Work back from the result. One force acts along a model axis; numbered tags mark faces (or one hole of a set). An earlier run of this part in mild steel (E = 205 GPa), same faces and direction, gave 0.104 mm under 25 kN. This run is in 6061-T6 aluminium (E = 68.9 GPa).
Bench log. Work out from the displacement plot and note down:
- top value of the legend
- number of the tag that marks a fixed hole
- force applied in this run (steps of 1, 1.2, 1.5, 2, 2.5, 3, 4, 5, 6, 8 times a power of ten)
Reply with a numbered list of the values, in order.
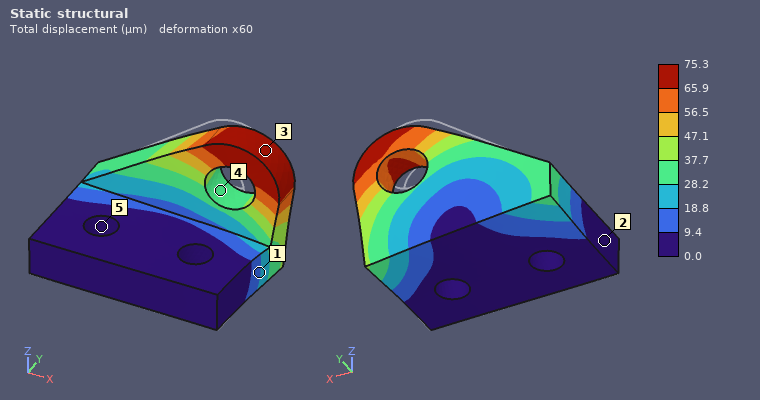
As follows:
1. 75.3 µm
2. 5
3. 6 kN
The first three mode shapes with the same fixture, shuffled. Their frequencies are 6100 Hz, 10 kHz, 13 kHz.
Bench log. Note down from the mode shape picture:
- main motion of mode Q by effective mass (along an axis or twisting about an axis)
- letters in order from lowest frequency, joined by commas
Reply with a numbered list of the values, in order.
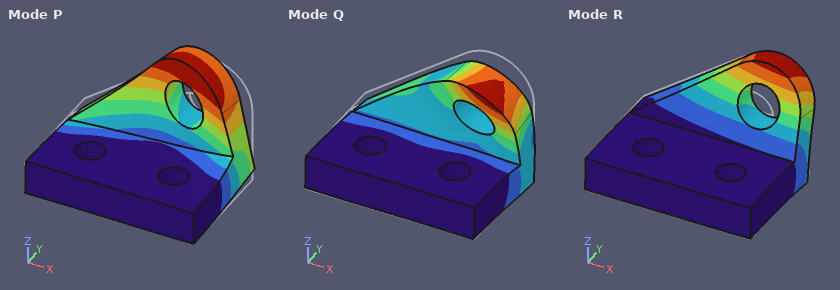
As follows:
1. along Z
2. R, P, Q
